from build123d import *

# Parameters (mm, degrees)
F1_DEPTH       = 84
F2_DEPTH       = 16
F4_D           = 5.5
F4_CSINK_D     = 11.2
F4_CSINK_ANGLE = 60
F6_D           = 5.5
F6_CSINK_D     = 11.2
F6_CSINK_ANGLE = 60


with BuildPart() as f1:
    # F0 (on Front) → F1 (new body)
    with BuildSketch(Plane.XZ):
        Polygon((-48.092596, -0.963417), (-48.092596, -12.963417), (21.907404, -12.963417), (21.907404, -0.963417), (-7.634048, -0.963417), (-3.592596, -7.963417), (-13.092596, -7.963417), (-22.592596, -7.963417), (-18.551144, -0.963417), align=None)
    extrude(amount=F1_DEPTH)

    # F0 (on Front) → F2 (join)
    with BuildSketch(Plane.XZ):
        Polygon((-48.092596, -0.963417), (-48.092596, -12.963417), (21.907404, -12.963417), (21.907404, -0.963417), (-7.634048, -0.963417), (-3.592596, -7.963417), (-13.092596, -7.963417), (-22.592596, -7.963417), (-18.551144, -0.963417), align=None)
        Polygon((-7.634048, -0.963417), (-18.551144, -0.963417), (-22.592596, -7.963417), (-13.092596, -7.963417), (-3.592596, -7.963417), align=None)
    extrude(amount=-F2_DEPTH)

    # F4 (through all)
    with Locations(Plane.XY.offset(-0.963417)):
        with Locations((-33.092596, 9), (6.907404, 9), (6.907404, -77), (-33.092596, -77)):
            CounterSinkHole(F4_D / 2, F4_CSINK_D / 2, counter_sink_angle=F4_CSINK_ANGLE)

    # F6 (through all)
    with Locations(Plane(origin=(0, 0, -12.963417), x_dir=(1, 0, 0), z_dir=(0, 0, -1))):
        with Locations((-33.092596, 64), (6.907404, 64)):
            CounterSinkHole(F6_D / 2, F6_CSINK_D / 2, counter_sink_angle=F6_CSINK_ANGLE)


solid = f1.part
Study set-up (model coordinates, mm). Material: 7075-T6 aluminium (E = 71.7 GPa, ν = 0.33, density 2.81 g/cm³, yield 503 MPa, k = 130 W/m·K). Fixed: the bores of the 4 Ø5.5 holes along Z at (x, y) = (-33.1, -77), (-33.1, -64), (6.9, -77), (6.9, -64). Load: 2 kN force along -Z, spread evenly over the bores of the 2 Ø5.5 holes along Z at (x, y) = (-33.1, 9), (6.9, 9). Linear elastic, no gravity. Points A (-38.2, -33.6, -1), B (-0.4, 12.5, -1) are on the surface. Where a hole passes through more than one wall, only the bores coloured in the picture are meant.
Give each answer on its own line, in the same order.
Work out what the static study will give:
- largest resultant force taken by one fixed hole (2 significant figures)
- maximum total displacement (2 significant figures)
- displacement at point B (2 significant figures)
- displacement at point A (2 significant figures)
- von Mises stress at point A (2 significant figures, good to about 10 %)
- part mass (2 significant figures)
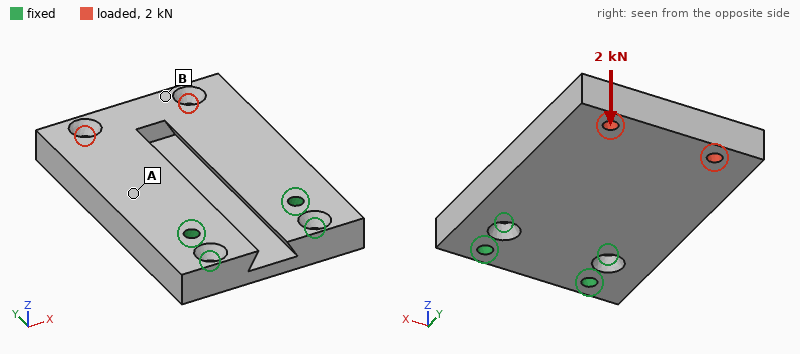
4.0 kN
0.58 mm
0.54 mm
0.14 mm
59 MPa
200 g
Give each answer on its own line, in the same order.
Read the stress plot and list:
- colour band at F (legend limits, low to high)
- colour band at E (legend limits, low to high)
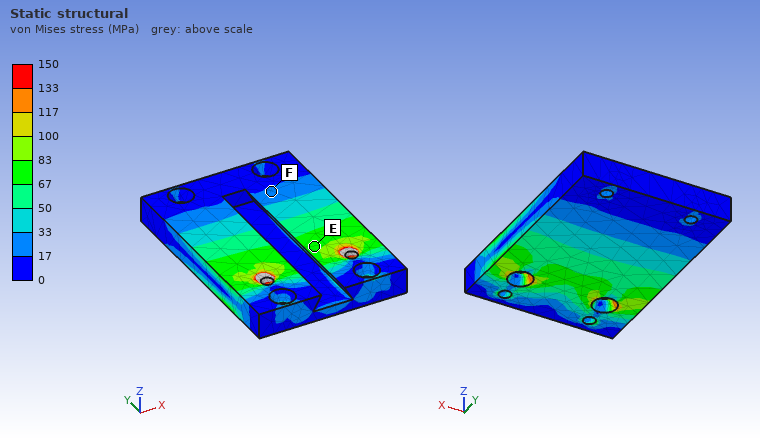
17 to 33 MPa
67 to 83 MPa
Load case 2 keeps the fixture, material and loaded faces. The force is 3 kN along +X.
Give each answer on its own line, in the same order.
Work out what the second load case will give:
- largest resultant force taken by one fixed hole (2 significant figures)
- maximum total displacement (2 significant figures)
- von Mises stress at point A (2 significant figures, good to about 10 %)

3.9 kN
53 µm
12 MPa
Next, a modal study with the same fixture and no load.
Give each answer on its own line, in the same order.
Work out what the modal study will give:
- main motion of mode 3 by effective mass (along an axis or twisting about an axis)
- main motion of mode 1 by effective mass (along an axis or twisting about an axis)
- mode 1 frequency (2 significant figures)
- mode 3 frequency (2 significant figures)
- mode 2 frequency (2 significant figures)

along X
along Z
1300 Hz
4900 Hz
3100 Hz
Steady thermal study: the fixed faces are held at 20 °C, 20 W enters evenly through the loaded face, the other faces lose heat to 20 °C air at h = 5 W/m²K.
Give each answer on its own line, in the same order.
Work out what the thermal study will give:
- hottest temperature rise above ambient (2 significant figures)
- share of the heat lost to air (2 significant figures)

18 K
3.7 %
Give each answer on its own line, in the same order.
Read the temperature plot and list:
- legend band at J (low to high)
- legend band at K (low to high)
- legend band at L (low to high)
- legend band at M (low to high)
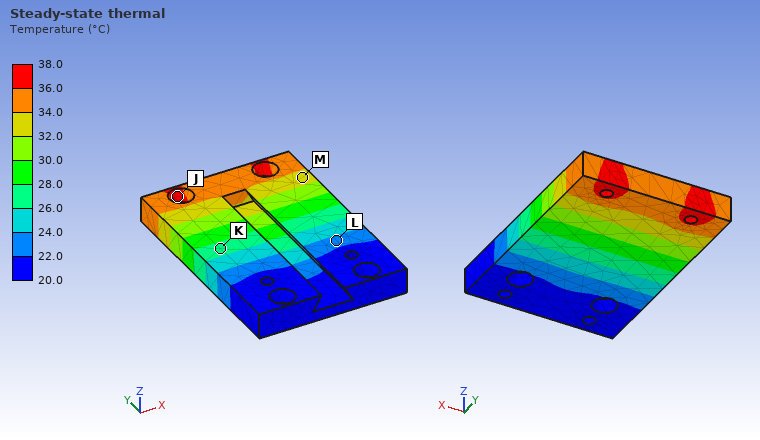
36.0 to 38.0 °C
26.0 to 28.0 °C
22.0 to 24.0 °C
32.0 to 34.0 °C
